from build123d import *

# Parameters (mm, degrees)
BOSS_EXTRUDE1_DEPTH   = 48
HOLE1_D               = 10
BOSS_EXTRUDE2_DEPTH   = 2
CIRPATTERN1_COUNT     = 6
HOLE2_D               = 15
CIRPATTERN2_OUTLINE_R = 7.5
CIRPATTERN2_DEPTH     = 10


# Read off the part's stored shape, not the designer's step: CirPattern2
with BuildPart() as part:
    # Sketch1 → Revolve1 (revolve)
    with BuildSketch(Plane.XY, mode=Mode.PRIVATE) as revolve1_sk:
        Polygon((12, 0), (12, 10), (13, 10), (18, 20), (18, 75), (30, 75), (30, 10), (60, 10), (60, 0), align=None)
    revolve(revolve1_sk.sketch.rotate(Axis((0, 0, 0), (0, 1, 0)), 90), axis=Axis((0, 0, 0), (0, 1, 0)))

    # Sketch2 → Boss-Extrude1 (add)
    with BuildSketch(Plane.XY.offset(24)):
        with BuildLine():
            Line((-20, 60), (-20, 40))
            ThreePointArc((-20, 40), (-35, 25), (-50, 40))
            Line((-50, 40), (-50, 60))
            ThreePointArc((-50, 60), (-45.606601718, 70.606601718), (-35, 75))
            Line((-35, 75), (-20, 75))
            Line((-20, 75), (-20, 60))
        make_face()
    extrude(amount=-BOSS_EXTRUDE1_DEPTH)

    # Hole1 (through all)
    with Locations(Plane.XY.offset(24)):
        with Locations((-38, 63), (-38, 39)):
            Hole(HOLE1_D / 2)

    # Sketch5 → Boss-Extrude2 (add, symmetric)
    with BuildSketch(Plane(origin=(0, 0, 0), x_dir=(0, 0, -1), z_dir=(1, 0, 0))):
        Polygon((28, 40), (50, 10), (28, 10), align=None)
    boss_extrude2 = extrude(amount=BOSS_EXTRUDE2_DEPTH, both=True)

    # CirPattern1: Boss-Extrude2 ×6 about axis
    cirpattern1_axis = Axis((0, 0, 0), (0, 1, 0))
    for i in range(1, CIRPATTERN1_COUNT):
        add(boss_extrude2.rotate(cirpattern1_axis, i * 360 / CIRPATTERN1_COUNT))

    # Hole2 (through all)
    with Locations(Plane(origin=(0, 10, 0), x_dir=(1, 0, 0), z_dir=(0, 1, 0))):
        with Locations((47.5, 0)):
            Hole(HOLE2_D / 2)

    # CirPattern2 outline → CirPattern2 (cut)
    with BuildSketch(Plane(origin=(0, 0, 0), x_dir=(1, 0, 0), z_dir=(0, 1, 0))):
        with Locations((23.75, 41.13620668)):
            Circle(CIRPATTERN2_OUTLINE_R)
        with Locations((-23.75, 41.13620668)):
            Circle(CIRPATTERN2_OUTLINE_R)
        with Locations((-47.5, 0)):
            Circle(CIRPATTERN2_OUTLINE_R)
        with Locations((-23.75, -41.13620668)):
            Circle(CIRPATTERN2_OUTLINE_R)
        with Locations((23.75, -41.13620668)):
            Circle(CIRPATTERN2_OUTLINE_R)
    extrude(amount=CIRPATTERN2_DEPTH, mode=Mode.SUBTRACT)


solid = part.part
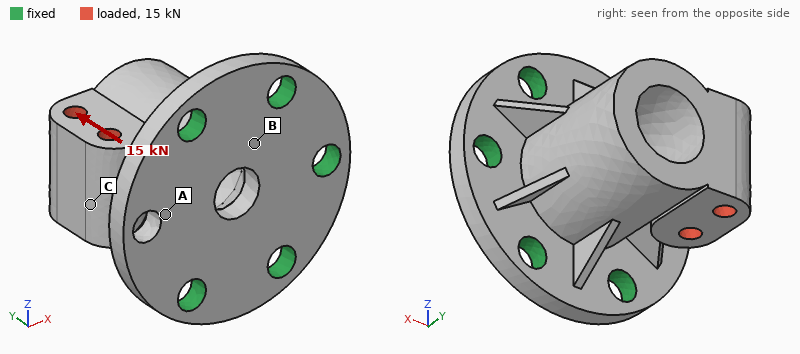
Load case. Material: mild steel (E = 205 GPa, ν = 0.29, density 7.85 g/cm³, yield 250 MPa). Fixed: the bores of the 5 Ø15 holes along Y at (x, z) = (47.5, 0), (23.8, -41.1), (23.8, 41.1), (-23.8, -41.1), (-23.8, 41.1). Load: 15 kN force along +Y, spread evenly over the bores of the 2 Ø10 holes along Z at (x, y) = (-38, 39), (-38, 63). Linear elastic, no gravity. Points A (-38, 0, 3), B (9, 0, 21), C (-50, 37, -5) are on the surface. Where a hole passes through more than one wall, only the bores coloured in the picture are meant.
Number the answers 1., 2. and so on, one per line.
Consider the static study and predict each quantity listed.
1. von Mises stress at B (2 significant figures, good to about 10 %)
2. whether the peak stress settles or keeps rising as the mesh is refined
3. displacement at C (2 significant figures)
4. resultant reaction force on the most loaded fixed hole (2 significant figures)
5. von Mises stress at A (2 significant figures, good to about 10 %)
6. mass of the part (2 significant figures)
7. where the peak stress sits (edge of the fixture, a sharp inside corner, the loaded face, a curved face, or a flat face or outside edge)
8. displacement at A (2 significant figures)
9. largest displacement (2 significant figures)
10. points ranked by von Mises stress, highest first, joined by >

1. 17 MPa
2. keeps rising
3. 33 µm
4. 9.1 kN
5. 32 MPa
6. 2.1 kg
7. edge of the fixture
8. 20 µm
9. 40 µm
10. A > B > C
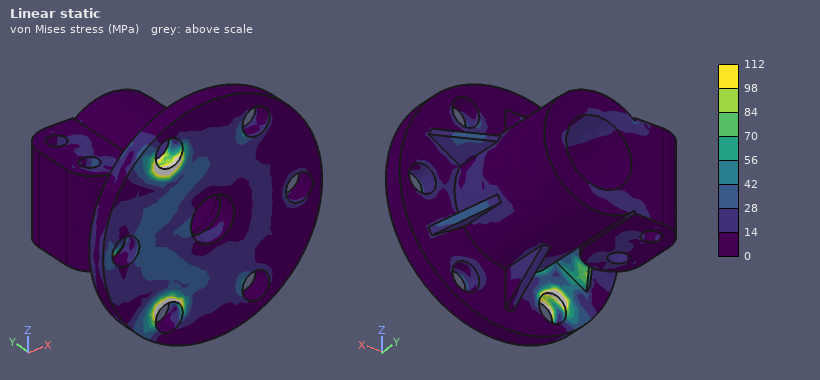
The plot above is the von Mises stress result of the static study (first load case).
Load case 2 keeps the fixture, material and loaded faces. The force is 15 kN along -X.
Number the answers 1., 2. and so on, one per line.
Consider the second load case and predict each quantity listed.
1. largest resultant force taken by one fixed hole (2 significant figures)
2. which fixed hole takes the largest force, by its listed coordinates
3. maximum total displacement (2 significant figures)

1. 7.5 kN
2. (47.5, 0)
3. 38 µm
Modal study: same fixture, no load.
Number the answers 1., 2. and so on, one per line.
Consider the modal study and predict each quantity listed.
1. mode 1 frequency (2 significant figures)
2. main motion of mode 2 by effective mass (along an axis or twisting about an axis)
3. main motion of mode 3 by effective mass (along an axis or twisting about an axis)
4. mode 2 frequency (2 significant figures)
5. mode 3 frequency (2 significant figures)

1. 3400 Hz
2. along Z
3. along Y
4. 4500 Hz
5. 7300 Hz
